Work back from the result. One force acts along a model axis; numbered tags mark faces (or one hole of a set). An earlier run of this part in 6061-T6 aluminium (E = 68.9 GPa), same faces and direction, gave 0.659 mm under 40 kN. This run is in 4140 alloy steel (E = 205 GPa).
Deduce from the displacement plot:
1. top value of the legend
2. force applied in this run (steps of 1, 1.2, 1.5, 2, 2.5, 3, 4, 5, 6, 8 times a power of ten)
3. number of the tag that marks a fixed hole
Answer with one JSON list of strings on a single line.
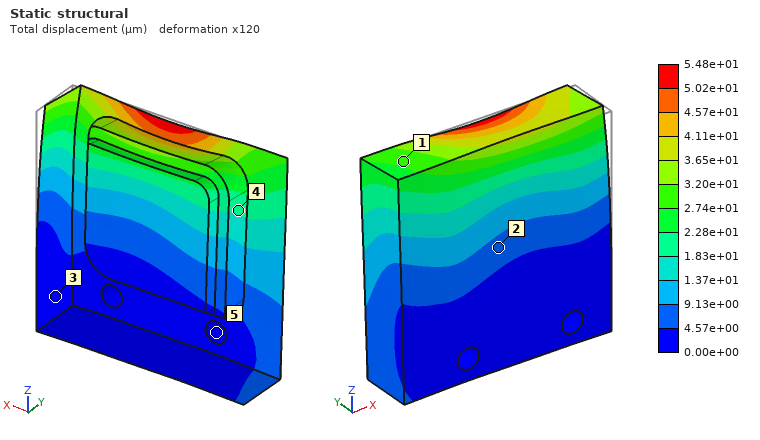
["5.48e+01 µm", "10 kN", "5"]
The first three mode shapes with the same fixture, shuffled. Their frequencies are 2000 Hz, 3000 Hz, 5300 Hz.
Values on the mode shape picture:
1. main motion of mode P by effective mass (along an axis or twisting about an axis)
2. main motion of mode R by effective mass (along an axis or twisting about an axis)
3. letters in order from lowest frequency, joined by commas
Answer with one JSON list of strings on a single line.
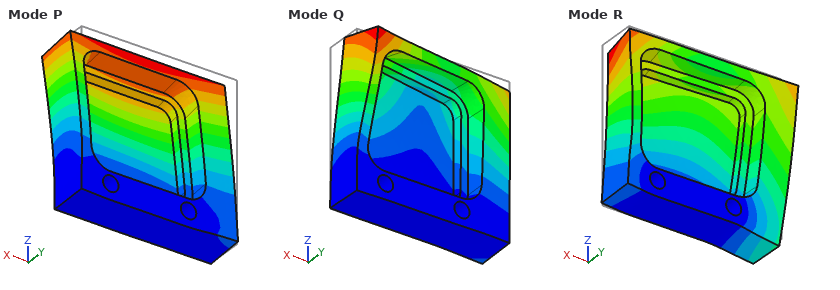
["along Y", "along X", "P, Q, R"]
